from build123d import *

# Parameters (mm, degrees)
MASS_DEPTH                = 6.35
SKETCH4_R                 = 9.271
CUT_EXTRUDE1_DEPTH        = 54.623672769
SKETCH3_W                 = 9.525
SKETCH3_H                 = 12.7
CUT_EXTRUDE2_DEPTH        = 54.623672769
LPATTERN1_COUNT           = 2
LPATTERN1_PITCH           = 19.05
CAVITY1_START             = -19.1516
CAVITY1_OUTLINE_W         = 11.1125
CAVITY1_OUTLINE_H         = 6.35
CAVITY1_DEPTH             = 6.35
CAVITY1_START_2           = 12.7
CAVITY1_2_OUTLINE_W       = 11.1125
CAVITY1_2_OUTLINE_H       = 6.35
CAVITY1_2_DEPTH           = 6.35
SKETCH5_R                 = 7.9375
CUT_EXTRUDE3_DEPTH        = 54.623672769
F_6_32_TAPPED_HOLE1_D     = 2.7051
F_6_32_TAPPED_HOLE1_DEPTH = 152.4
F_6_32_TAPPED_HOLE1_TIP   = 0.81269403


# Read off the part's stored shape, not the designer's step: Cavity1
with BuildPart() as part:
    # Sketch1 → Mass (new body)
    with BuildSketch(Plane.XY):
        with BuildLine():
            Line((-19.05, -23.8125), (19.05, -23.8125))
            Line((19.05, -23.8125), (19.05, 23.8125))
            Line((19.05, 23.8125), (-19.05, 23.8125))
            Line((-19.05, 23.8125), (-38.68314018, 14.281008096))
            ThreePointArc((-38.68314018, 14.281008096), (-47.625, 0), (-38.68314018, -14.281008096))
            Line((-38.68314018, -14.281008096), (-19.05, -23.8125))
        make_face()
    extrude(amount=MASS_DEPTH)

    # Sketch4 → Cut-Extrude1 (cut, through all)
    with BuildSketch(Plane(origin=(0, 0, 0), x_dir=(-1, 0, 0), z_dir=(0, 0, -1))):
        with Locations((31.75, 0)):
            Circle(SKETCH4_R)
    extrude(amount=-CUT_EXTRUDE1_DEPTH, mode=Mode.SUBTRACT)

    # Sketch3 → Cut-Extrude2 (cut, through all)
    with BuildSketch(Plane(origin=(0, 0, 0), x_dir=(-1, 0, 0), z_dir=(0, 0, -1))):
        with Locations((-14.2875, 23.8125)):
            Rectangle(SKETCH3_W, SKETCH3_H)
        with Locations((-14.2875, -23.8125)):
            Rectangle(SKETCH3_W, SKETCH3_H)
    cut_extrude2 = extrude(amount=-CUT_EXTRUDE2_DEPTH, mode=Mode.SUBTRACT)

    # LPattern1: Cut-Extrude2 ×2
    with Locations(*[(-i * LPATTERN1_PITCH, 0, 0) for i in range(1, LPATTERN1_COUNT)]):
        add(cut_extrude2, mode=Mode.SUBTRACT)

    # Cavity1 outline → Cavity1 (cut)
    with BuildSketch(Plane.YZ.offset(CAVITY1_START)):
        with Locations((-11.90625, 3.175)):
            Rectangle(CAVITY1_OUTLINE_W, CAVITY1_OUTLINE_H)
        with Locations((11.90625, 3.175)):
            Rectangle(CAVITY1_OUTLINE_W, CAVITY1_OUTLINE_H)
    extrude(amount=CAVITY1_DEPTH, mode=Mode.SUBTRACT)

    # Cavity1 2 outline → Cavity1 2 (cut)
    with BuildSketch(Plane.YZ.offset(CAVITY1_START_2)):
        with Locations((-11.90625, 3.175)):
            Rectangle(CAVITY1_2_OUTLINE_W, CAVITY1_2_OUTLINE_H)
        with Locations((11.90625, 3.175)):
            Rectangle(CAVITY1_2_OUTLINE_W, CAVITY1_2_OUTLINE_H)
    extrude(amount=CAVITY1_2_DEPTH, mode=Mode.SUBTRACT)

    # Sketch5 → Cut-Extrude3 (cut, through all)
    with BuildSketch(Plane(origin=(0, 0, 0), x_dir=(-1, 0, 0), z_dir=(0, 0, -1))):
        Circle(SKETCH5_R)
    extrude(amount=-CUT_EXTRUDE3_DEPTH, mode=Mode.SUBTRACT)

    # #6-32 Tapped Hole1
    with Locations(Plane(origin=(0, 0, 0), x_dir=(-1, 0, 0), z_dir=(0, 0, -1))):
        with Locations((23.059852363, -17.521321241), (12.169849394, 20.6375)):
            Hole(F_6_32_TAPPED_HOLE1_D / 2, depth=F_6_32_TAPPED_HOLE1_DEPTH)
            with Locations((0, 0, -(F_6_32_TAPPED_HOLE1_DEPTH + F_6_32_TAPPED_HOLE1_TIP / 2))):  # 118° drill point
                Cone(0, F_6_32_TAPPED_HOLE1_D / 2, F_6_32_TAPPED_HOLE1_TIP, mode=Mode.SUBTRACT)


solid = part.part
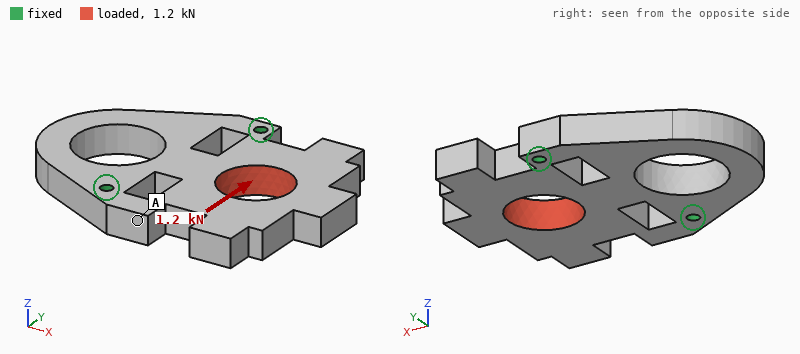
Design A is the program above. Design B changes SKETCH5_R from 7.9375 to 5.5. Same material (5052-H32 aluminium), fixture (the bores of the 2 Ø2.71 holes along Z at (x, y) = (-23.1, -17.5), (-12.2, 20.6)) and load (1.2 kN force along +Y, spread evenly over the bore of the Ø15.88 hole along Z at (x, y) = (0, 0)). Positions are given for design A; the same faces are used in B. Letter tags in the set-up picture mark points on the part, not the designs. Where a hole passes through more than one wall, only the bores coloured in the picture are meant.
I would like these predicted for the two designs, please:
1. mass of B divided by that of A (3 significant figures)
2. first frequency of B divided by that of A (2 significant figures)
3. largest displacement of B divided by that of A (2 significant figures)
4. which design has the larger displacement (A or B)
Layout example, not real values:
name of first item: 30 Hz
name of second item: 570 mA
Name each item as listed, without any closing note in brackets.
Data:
mass of B divided by that of A: 1.06
first frequency of B divided by that of A: 0.99
largest displacement of B divided by that of A: 0.75
which design has the larger displacement: A
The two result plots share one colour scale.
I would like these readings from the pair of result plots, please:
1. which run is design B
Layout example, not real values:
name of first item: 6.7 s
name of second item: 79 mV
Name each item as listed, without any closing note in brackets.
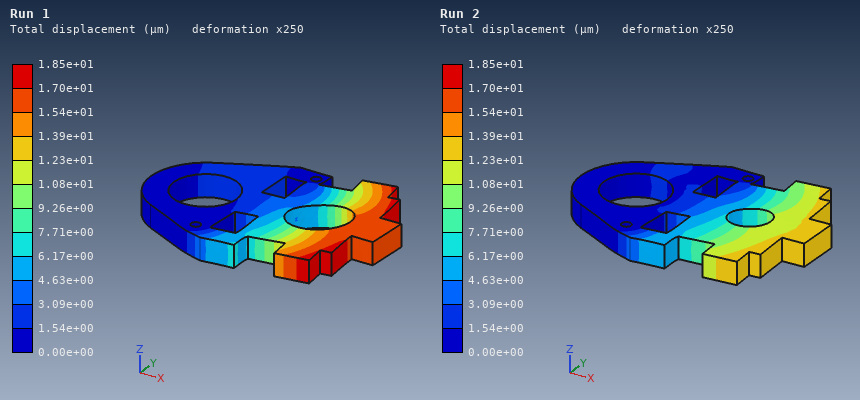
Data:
which run is design B: Run 2
